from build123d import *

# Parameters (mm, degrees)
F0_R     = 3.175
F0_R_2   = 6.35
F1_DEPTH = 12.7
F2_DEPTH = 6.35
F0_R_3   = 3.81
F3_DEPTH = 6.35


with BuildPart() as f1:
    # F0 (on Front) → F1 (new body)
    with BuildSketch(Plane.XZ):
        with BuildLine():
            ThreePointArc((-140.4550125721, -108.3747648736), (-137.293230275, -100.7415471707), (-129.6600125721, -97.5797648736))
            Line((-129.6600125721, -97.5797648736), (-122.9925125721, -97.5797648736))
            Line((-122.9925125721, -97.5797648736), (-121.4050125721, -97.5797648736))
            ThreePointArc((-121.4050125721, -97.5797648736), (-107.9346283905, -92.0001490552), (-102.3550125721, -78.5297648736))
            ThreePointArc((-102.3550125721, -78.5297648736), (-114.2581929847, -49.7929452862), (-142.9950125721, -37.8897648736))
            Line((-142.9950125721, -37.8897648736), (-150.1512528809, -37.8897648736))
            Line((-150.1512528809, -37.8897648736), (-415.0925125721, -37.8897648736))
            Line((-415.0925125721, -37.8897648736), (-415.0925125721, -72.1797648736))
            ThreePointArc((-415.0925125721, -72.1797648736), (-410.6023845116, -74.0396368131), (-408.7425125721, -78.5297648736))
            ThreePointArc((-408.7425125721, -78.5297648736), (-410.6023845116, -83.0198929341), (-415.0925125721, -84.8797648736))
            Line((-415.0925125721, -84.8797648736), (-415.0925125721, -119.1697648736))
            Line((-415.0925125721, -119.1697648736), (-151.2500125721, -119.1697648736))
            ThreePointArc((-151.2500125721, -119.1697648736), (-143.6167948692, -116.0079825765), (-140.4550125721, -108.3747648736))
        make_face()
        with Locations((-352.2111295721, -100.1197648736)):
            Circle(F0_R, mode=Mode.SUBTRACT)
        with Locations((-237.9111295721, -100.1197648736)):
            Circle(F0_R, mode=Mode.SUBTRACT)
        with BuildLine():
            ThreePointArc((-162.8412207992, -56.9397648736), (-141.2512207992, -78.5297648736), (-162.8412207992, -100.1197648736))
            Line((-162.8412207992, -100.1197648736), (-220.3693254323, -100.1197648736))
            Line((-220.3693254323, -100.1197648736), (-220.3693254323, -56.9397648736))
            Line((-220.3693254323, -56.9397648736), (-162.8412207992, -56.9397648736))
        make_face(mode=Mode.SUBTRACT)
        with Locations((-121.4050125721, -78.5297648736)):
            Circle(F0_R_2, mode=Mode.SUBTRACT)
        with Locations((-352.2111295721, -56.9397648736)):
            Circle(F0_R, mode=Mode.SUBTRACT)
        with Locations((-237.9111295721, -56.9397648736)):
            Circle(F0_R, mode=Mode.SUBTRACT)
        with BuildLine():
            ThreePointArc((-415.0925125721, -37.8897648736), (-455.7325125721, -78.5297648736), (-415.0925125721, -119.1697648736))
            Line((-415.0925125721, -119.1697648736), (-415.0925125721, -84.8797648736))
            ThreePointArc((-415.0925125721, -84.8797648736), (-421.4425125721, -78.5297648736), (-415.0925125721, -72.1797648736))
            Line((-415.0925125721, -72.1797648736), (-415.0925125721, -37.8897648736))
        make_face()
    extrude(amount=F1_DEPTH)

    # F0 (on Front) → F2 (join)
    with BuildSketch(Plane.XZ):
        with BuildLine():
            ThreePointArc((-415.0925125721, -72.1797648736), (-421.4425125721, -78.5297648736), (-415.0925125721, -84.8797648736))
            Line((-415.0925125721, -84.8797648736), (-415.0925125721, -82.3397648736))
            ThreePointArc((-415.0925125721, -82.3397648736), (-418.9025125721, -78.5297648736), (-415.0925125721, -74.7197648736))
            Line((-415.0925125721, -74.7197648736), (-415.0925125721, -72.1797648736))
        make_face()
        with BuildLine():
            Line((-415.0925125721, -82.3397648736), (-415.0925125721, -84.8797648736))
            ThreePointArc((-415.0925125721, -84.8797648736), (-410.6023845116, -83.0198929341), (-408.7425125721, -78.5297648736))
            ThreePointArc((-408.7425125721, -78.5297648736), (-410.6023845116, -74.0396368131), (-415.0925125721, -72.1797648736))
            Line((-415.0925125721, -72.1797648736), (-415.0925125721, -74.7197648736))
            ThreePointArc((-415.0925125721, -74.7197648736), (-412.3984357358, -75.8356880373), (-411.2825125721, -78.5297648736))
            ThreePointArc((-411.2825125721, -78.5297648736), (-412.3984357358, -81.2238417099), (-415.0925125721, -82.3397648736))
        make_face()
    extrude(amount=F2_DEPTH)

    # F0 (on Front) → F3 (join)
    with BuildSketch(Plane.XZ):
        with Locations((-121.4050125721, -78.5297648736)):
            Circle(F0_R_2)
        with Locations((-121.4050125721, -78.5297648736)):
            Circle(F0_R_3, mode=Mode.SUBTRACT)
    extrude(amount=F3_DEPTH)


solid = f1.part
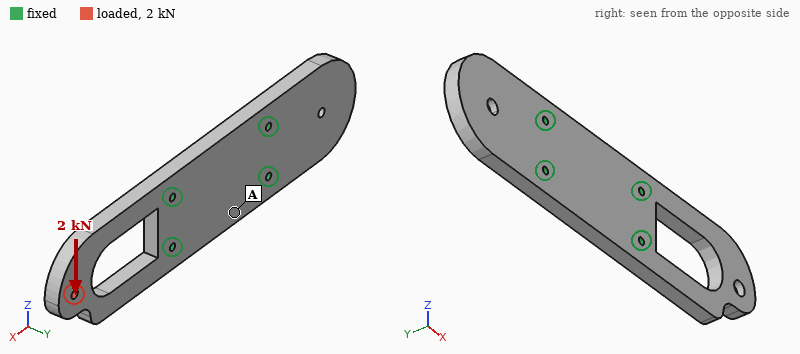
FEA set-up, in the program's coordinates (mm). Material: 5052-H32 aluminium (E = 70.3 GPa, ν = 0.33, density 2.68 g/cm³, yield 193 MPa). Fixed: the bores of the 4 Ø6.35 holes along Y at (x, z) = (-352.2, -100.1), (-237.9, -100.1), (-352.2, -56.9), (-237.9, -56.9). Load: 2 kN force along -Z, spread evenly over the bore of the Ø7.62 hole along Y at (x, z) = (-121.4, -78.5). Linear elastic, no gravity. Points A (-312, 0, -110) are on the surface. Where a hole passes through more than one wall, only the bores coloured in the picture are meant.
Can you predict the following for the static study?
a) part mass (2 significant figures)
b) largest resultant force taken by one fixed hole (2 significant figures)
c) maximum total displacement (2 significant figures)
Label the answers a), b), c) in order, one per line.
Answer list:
a) 790 g
b) 3.1 kN
c) 0.19 mm
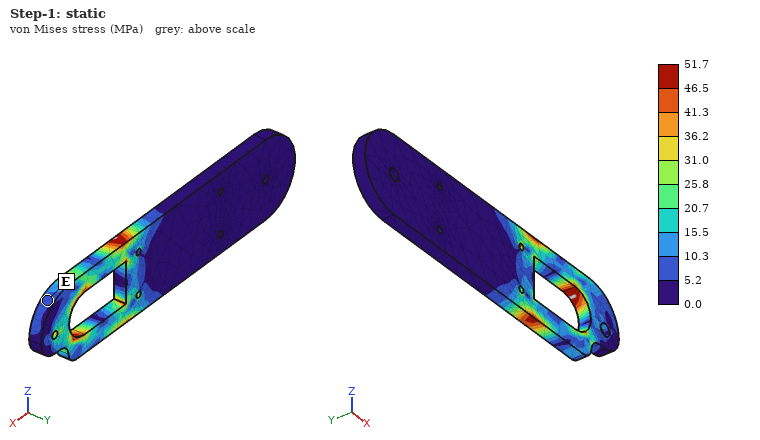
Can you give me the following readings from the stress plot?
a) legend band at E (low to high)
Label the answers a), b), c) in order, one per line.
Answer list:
a) 5.2 to 10.3 MPa
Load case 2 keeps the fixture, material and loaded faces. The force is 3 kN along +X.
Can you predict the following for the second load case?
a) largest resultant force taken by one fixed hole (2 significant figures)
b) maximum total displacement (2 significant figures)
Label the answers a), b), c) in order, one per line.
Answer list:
a) 1.3 kN
b) 0.19 mm
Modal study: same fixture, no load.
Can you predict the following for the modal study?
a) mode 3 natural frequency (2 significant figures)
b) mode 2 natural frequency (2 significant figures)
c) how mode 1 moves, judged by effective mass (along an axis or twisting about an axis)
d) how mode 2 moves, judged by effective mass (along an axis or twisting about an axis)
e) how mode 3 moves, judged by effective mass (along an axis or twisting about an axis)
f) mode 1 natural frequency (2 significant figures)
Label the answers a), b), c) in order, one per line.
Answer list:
a) 1600 Hz
b) 1100 Hz
c) along Y
d) along Y
e) along Z
f) 550 Hz
